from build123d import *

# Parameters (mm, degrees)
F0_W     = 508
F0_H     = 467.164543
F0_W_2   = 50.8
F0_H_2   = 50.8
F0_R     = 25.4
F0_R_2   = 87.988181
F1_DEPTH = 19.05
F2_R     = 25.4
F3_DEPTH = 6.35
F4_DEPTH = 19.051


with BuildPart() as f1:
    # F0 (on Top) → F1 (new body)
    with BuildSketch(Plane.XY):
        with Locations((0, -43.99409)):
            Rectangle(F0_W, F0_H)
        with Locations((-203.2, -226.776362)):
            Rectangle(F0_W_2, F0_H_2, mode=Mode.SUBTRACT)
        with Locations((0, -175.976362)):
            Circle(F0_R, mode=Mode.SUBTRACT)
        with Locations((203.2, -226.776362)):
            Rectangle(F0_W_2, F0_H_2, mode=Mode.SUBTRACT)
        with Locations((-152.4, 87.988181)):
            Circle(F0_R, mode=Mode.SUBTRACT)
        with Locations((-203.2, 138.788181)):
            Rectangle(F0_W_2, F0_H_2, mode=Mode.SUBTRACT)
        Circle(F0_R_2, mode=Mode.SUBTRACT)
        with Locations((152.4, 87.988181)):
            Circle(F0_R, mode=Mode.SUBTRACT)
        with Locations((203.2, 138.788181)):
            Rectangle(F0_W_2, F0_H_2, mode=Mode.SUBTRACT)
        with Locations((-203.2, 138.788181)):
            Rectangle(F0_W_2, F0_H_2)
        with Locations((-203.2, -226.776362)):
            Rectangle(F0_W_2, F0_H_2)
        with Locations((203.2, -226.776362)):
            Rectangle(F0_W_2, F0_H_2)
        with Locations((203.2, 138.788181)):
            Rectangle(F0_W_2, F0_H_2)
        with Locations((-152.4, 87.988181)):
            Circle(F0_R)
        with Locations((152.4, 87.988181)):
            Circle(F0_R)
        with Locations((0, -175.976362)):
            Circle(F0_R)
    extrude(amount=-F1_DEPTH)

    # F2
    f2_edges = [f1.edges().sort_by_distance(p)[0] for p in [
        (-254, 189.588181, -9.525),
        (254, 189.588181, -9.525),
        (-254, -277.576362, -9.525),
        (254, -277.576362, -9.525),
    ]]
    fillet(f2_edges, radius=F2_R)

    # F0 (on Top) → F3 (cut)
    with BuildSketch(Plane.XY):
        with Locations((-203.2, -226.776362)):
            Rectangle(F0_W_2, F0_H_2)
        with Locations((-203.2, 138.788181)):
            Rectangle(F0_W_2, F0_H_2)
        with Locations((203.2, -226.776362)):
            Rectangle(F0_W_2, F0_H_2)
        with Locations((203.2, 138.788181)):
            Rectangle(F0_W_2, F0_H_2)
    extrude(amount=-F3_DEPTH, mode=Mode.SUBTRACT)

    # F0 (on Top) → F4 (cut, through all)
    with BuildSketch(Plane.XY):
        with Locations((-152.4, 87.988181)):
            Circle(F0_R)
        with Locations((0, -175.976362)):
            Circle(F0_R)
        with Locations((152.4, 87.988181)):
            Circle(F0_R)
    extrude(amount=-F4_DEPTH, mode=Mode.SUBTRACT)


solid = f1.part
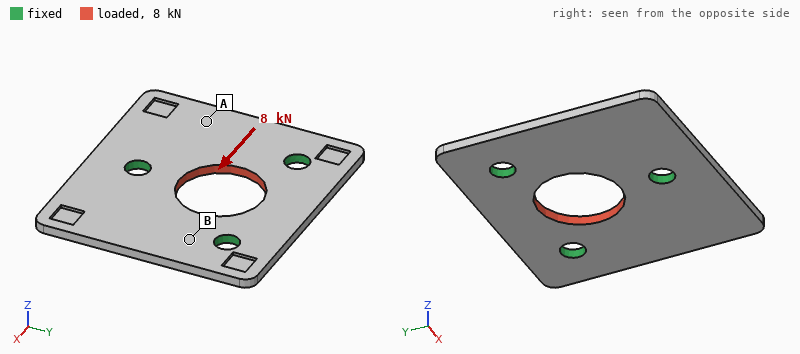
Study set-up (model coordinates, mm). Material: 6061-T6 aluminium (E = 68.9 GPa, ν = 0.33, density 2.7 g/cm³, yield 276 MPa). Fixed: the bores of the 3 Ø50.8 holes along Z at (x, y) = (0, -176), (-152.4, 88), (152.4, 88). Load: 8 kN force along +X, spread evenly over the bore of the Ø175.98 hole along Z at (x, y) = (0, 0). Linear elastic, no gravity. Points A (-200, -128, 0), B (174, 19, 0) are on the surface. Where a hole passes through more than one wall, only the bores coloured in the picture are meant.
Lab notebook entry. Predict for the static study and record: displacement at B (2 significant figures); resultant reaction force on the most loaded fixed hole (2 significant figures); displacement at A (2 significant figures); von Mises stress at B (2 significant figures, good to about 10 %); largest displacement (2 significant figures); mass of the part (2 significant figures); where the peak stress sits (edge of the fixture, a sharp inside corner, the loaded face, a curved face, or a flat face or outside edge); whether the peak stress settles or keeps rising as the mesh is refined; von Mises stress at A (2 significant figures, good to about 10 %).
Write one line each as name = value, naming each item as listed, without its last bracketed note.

displacement at B = 1.1 µm
resultant reaction force on the most loaded fixed hole = 2.9 kN
displacement at A = 1.4 µm
von Mises stress at B = 0.74 MPa
largest displacement = 2.5 µm
mass of the part = 10 kg
where the peak stress sits = edge of the fixture
whether the peak stress settles or keeps rising as the mesh is refined = keeps rising
von Mises stress at A = 0.33 MPa
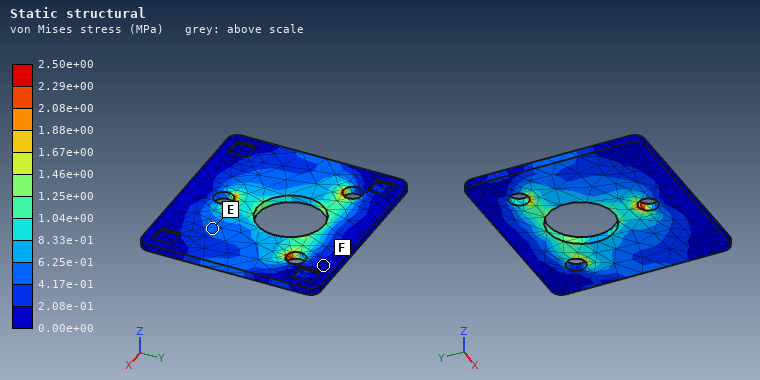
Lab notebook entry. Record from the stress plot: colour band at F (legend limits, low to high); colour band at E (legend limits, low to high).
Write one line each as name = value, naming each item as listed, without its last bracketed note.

colour band at F = 0.00e+00 to 2.08e-01 MPa
colour band at E = 4.17e-01 to 6.25e-01 MPa
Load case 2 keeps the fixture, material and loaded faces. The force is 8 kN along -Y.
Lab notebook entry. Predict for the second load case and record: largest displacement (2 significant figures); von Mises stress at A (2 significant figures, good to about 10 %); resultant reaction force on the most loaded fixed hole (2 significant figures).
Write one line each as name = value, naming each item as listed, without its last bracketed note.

largest displacement = 3.9 µm
von Mises stress at A = 0.22 MPa
resultant reaction force on the most loaded fixed hole = 2.8 kN
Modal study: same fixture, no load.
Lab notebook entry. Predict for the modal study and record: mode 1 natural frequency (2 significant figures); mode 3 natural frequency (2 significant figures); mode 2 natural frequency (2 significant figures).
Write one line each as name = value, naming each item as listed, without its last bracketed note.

mode 1 natural frequency = 370 Hz
mode 3 natural frequency = 920 Hz
mode 2 natural frequency = 380 Hz
